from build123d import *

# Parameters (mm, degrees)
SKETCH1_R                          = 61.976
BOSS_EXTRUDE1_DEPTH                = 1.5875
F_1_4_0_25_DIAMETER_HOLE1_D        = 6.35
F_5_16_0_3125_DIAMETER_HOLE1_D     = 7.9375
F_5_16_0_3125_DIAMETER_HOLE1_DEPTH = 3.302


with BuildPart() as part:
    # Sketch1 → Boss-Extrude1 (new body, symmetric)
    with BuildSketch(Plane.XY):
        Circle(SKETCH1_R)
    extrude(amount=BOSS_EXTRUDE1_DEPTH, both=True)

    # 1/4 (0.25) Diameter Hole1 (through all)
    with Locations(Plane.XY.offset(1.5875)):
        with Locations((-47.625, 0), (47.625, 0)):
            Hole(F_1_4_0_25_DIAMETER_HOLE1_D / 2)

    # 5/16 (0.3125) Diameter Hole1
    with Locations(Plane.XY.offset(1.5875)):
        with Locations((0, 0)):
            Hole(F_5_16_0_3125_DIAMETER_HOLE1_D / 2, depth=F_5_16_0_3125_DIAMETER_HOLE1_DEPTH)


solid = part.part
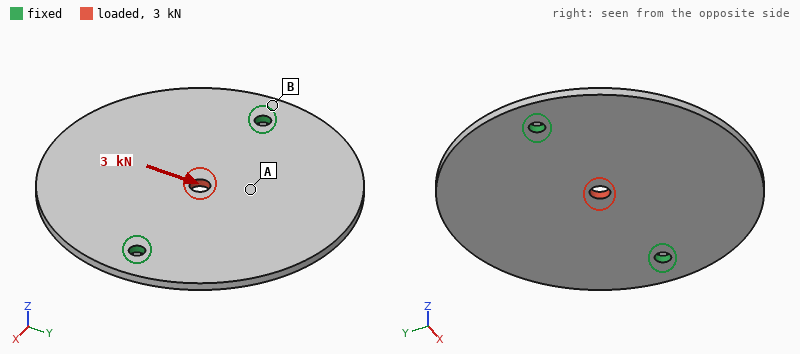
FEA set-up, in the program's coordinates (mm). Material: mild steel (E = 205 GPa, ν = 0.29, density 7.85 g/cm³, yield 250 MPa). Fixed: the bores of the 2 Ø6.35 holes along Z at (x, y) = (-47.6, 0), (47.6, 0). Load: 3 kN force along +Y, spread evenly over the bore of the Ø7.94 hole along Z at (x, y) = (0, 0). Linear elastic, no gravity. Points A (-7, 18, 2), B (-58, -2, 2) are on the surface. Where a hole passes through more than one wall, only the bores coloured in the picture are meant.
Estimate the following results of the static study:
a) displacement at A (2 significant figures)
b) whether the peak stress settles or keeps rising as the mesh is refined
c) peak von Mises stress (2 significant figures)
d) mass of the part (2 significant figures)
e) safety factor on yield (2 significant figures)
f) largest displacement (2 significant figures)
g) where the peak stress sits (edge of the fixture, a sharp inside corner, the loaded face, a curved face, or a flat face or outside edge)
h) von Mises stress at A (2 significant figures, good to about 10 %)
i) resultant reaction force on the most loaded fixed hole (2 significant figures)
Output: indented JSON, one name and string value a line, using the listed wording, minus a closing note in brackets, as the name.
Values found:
{
  "displacement at A": "4.0 µm",
  "whether the peak stress settles or keeps rising as the mesh is refined": "settles",
  "peak von Mises stress": "66 MPa",
  "mass of the part": "300 g",
  "safety factor on yield": "3.8",
  "largest displacement": "5.9 µm",
  "where the peak stress sits": "the loaded face",
  "von Mises stress at A": "14 MPa",
  "resultant reaction force on the most loaded fixed hole": "1.5 kN"
}
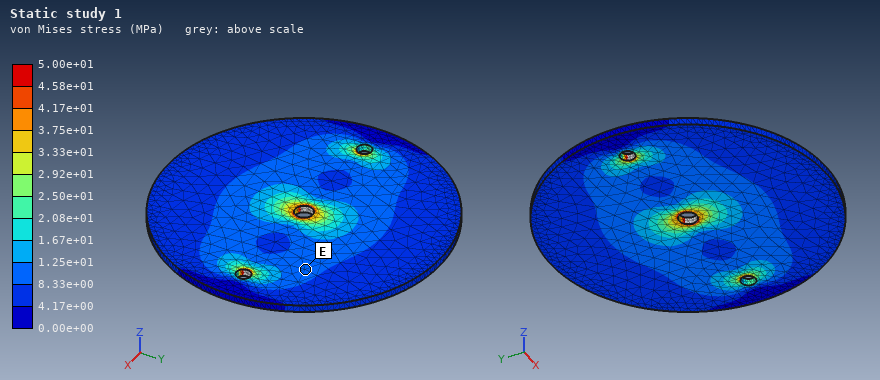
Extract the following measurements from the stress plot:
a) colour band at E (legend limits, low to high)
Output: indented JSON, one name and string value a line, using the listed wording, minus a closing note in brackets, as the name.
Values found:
{
  "colour band at E": "8.33e+00 to 1.25e+01 MPa"
}
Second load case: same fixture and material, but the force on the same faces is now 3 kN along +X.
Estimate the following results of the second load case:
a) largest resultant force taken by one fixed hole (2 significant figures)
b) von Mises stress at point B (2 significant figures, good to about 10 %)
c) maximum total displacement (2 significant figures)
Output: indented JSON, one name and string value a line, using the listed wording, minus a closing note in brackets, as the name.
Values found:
{
  "largest resultant force taken by one fixed hole": "1.5 kN",
  "von Mises stress at point B": "8.1 MPa",
  "maximum total displacement": "4.4 µm"
}
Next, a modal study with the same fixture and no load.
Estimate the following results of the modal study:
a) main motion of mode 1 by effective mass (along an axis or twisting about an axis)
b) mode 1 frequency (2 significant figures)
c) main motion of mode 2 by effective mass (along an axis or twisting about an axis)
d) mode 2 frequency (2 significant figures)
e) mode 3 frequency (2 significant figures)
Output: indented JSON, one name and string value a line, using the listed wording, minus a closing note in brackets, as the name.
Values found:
{
  "main motion of mode 1 by effective mass": "twisting about X",
  "mode 1 frequency": "620 Hz",
  "main motion of mode 2 by effective mass": "along Z",
  "mode 2 frequency": "810 Hz",
  "mode 3 frequency": "1800 Hz"
}
